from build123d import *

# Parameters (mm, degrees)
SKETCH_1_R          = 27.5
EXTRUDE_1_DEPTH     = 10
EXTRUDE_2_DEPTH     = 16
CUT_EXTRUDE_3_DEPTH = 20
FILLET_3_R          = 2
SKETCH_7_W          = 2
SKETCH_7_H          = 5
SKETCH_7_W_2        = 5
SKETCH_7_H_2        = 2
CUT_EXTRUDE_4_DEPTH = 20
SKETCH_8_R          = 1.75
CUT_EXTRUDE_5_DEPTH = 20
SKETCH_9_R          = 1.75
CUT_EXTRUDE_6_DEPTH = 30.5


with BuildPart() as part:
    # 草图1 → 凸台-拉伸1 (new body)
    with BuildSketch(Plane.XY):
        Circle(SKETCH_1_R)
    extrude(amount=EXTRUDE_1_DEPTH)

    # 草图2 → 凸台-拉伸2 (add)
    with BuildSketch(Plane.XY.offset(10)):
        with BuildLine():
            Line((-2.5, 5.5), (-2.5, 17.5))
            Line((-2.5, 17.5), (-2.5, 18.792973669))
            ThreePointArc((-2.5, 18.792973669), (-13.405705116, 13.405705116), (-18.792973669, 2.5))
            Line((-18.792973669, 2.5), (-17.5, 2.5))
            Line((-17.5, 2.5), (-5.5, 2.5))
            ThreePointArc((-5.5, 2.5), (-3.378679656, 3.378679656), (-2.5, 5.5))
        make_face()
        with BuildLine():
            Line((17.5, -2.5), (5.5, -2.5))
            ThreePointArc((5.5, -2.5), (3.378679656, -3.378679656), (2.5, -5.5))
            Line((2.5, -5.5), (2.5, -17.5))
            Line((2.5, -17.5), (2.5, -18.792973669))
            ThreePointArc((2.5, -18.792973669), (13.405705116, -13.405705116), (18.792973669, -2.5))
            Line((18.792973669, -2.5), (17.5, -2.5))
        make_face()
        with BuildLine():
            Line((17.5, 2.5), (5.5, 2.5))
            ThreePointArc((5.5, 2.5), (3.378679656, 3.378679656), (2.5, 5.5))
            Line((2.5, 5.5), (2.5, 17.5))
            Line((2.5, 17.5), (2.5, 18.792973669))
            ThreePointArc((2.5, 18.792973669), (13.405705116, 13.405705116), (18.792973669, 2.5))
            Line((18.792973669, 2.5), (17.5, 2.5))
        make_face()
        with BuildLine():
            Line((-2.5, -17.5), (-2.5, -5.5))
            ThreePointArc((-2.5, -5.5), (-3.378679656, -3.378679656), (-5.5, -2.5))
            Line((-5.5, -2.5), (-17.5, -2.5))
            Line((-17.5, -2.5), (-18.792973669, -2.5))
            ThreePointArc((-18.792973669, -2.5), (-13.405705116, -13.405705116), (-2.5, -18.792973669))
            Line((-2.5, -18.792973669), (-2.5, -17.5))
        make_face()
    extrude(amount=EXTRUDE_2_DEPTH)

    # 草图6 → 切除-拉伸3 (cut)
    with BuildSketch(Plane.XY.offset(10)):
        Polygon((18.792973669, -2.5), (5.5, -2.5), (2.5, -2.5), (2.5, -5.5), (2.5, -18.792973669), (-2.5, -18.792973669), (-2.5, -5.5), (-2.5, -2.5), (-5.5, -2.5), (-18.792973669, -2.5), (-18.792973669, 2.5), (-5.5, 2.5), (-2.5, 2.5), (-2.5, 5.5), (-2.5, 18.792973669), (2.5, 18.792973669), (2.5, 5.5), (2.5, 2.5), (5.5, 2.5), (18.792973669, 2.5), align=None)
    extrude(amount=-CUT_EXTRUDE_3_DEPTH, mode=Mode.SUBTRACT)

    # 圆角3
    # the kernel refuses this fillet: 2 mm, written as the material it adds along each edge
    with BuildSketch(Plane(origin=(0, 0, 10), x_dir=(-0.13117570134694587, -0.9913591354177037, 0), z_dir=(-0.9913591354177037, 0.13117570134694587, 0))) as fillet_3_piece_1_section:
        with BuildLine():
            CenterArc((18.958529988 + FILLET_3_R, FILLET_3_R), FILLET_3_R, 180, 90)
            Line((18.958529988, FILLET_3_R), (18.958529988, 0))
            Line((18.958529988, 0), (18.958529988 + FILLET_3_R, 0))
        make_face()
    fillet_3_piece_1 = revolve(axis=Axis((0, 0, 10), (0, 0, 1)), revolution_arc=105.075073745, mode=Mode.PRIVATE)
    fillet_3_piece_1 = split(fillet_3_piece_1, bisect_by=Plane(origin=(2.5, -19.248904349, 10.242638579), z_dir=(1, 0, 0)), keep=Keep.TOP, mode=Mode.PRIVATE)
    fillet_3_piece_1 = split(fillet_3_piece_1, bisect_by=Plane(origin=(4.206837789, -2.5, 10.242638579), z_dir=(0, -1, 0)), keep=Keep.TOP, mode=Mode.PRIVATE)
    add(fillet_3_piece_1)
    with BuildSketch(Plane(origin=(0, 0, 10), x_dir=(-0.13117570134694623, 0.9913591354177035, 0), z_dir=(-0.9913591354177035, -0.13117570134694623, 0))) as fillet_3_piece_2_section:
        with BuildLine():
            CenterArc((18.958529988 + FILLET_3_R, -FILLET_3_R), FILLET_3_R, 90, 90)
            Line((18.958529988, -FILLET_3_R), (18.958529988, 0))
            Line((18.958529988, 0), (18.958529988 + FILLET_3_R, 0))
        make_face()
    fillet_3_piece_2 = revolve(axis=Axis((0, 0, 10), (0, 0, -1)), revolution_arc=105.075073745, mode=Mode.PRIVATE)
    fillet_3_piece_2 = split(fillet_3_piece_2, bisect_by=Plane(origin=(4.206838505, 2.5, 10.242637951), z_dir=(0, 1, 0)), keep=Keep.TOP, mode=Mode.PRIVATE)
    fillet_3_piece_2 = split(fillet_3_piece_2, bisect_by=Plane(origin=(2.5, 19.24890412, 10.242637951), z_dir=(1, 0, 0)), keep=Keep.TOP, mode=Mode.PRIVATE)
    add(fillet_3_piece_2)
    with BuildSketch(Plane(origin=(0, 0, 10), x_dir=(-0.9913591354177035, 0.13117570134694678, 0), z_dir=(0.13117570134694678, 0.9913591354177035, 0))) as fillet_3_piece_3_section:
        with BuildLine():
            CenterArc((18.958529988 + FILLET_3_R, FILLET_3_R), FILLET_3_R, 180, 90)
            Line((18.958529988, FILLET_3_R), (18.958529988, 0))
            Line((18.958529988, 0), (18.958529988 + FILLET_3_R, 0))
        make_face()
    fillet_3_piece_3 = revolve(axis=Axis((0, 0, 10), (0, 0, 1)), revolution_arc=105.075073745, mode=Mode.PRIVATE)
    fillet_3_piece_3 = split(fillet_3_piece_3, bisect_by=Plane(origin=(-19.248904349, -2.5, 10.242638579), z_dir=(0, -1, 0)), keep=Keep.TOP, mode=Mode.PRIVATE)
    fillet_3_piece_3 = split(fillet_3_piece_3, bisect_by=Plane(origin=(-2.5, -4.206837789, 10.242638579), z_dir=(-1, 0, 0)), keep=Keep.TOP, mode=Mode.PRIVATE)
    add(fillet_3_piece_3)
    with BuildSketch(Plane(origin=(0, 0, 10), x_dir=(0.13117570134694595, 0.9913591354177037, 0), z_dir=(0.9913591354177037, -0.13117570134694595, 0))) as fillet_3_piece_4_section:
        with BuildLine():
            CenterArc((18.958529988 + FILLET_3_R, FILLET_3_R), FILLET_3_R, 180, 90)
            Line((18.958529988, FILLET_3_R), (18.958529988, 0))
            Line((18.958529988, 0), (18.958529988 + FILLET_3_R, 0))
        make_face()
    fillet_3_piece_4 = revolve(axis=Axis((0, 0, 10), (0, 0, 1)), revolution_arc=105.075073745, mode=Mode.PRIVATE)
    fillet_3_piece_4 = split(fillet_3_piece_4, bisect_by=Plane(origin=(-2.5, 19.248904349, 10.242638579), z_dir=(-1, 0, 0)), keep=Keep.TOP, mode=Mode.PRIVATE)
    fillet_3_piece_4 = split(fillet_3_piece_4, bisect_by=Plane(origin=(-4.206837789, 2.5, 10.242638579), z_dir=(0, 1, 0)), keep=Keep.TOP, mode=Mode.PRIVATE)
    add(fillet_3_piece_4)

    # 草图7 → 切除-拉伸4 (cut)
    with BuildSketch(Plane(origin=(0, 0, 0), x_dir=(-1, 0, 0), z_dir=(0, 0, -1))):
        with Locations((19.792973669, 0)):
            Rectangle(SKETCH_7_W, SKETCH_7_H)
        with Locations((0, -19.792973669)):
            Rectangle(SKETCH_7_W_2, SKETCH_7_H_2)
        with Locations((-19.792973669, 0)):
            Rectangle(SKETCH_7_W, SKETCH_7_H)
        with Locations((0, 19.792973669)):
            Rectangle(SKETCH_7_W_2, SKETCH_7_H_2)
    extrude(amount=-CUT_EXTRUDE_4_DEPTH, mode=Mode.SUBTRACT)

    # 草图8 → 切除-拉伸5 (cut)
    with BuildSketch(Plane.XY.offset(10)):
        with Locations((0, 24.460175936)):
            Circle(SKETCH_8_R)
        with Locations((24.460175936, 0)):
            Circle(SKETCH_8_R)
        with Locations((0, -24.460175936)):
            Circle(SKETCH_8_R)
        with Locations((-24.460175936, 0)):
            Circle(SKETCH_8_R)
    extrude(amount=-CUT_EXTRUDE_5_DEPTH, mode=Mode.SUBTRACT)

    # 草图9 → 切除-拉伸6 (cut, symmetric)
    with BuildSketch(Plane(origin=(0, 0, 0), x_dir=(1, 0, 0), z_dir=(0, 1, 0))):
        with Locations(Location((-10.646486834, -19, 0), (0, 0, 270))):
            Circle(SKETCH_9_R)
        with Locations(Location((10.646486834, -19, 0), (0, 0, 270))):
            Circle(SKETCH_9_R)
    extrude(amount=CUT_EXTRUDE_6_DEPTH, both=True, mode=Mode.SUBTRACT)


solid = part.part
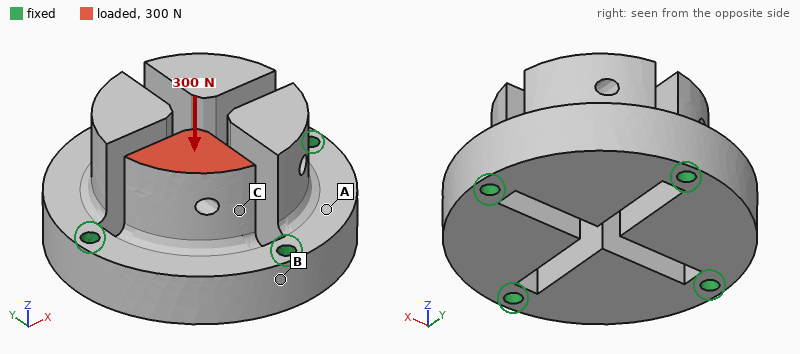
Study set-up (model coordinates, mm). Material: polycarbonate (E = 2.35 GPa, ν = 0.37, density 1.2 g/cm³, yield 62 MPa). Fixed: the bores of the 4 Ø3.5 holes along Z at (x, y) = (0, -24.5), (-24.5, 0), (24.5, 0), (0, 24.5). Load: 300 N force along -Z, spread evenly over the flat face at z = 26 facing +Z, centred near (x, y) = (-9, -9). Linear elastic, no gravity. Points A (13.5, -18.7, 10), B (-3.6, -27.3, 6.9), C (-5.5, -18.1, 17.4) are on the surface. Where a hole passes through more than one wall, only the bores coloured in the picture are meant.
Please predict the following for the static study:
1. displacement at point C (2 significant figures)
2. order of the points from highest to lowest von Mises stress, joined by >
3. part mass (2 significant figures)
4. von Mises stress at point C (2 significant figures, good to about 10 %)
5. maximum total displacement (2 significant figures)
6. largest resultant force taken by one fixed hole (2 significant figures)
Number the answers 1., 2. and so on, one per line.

1. 0.15 mm
2. B > C > A
3. 38 g
4. 2.4 MPa
5. 0.31 mm
6. 150 N
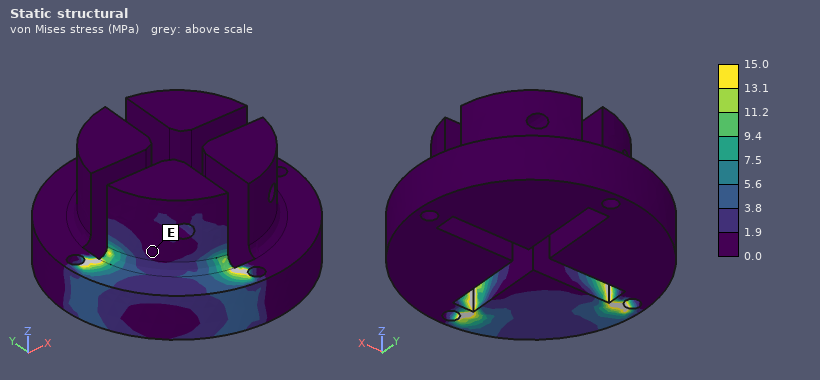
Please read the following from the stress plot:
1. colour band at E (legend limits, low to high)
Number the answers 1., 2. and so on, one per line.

1. 0.0 to 1.9 MPa
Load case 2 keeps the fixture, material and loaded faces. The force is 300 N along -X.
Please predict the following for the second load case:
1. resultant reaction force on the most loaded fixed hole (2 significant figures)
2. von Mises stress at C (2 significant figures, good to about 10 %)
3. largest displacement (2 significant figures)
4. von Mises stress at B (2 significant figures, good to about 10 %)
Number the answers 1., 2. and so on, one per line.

1. 220 N
2. 4.0 MPa
3. 0.81 mm
4. 12 MPa
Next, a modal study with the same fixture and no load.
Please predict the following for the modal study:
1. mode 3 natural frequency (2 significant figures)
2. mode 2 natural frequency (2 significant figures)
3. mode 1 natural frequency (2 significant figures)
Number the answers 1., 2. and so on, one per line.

1. 2000 Hz
2. 2000 Hz
3. 1900 Hz
